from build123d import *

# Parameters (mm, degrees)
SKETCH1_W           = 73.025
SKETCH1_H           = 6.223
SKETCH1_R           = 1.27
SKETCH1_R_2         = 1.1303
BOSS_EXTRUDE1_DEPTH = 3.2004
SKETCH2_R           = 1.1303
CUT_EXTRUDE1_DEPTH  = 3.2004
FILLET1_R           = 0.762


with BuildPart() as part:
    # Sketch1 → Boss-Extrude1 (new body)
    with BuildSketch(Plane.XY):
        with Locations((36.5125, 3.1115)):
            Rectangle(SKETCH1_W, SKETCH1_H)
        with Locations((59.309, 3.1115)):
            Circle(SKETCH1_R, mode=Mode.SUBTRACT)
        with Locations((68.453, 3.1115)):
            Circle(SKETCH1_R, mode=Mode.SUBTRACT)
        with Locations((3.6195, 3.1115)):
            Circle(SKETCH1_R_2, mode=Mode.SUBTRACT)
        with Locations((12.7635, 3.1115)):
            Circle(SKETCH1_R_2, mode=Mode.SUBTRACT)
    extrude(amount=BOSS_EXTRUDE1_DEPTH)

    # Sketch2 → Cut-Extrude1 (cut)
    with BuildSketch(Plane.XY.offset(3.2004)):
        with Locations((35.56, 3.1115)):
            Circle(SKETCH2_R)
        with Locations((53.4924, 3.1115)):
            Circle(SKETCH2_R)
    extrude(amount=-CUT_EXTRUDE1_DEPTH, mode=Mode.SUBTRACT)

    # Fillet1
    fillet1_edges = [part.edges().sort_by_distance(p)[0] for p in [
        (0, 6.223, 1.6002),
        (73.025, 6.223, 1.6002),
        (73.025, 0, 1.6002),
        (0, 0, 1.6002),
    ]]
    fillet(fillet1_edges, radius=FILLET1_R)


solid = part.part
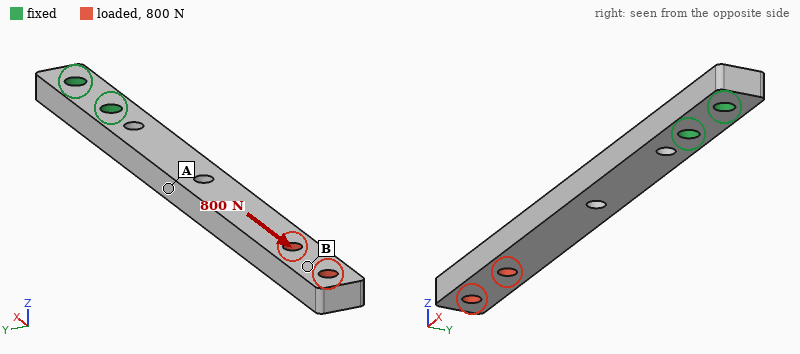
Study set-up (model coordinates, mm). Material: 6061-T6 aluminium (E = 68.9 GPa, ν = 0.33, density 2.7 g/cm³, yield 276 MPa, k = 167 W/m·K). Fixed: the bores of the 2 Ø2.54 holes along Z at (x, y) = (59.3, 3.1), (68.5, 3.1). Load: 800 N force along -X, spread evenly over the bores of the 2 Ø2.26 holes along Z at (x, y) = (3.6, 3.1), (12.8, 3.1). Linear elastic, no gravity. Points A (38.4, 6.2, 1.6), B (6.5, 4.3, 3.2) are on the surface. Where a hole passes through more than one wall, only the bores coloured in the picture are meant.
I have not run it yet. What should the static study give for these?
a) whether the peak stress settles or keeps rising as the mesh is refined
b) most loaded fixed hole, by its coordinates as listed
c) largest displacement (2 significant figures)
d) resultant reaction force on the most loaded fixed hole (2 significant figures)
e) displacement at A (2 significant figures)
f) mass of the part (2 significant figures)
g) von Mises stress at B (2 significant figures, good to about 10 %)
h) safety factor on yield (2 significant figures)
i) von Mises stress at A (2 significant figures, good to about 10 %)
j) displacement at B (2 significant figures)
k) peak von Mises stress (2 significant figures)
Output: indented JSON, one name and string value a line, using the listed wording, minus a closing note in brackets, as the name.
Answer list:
{
  "whether the peak stress settles or keeps rising as the mesh is refined": "settles",
  "most loaded fixed hole, by its coordinates as listed": "(59.3, 3.1)",
  "largest displacement": "34 µm",
  "resultant reaction force on the most loaded fixed hole": "760 N",
  "displacement at A": "14 µm",
  "mass of the part": "3.7 g",
  "von Mises stress at B": "20 MPa",
  "safety factor on yield": "1.9",
  "von Mises stress at A": "54 MPa",
  "displacement at B": "33 µm",
  "peak von Mises stress": "140 MPa"
}
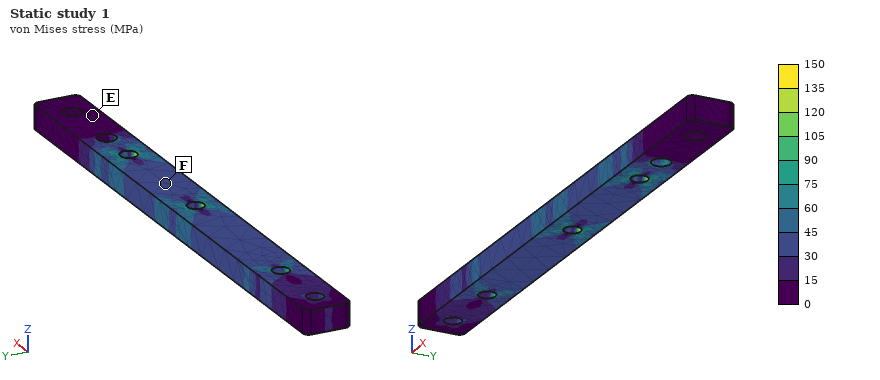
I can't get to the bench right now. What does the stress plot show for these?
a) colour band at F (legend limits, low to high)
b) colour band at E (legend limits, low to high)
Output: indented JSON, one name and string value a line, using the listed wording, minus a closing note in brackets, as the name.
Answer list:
{
  "colour band at F": "30 to 45 MPa",
  "colour band at E": "0 to 15 MPa"
}
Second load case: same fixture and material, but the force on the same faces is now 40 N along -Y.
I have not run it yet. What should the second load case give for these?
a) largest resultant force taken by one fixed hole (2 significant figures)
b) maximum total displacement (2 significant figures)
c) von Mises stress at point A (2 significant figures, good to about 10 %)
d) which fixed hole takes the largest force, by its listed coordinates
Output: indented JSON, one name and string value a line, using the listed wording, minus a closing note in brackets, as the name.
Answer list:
{
  "largest resultant force taken by one fixed hole": "110 N",
  "maximum total displacement": "0.54 mm",
  "von Mises stress at point A": "61 MPa",
  "which fixed hole takes the largest force, by its listed coordinates": "(59.3, 3.1)"
}
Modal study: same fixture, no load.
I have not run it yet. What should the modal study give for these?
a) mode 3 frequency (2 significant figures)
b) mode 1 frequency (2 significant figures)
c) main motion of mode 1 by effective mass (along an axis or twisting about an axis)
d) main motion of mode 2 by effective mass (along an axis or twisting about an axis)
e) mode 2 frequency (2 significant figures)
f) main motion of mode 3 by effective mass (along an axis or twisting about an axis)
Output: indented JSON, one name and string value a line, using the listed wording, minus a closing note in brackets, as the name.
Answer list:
{
  "mode 3 frequency": "4600 Hz",
  "mode 1 frequency": "740 Hz",
  "main motion of mode 1 by effective mass": "along Z",
  "main motion of mode 2 by effective mass": "along Y",
  "mode 2 frequency": "1400 Hz",
  "main motion of mode 3 by effective mass": "along Z"
}
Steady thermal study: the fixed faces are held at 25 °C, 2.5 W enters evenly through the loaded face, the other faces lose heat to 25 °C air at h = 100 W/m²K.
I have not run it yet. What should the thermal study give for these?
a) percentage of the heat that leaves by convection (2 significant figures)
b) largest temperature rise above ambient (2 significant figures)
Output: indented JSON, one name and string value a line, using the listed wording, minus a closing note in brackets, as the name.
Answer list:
{
  "percentage of the heat that leaves by convection": "55 %",
  "largest temperature rise above ambient": "24 K"
}
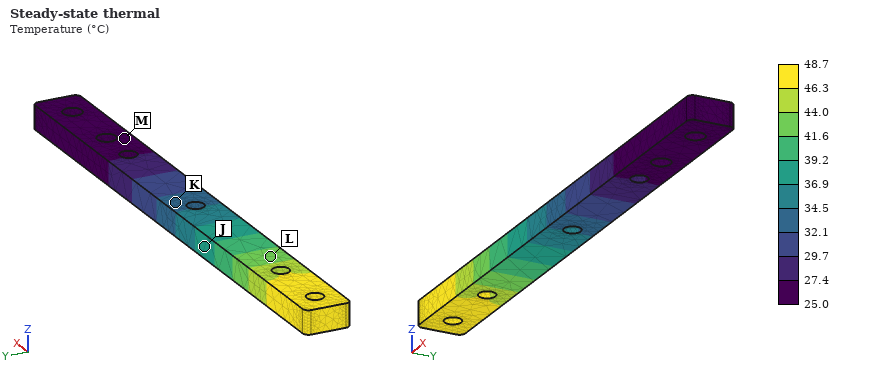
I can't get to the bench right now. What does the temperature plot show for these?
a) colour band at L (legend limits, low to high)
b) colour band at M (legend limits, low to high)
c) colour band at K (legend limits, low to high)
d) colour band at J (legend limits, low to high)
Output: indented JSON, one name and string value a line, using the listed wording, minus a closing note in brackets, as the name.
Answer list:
{
  "colour band at L": "41.6 to 44.0 °C",
  "colour band at M": "25.0 to 27.4 °C",
  "colour band at K": "32.1 to 34.5 °C",
  "colour band at J": "36.9 to 39.2 °C"
}
